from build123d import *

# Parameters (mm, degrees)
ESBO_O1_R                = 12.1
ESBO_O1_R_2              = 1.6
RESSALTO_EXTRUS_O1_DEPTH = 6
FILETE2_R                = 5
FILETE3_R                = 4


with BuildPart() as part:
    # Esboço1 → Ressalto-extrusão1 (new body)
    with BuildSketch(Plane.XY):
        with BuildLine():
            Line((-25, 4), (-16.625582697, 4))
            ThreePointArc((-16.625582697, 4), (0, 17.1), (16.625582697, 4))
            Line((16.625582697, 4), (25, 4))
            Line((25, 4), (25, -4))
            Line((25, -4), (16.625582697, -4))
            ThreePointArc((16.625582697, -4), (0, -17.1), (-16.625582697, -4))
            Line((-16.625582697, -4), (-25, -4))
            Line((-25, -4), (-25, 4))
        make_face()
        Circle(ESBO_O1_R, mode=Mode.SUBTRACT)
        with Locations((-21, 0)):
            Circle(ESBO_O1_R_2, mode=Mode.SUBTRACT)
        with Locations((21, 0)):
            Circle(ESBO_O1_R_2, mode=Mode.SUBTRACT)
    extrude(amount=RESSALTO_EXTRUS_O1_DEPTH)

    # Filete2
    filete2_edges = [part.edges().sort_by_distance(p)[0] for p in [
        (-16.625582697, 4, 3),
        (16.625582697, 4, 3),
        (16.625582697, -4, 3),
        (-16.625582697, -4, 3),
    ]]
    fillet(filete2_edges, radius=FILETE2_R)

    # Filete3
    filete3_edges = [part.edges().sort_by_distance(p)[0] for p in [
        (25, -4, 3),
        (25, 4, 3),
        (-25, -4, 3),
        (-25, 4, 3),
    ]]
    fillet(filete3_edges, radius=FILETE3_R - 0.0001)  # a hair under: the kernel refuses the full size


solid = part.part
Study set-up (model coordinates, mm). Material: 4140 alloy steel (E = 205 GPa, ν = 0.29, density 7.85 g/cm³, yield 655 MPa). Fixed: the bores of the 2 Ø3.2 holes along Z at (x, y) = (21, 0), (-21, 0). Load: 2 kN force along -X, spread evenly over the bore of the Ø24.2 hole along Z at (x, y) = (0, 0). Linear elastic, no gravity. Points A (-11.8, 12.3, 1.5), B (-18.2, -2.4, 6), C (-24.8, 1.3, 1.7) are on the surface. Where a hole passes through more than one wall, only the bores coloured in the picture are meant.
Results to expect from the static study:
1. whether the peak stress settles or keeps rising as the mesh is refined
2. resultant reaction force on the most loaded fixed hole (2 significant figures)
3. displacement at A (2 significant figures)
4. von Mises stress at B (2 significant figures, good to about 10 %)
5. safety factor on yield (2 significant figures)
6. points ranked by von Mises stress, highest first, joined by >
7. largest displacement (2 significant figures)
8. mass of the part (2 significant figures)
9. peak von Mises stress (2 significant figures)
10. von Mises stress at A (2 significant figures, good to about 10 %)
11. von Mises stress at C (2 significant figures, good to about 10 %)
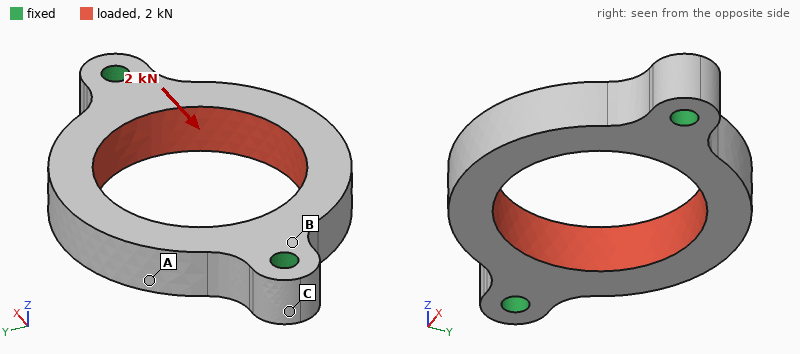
settles
1.0 kN
3.5 µm
23 MPa
12
B > A > C
3.8 µm
27 g
54 MPa
15 MPa
4.9 MPa
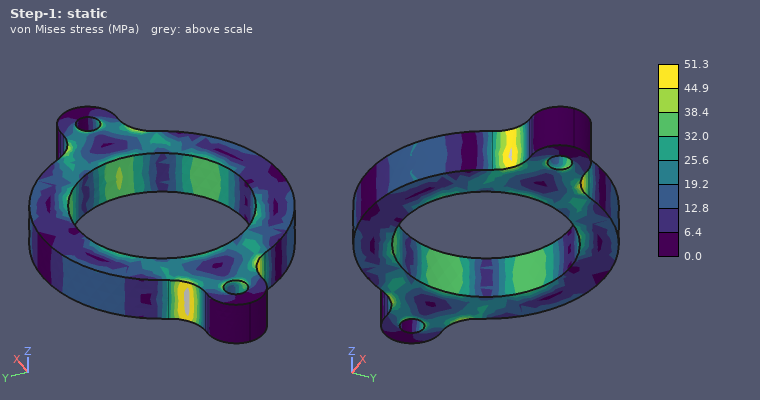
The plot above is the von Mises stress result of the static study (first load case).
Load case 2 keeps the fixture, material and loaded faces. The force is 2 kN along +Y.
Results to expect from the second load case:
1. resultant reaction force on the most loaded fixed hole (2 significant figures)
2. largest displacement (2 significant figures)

1.0 kN
3.2 µm
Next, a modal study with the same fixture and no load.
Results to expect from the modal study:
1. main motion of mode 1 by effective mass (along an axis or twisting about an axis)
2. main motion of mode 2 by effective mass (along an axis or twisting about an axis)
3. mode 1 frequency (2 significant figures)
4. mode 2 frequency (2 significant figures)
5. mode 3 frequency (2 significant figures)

twisting about X
along Z
8700 Hz
11 kHz
20 kHz
